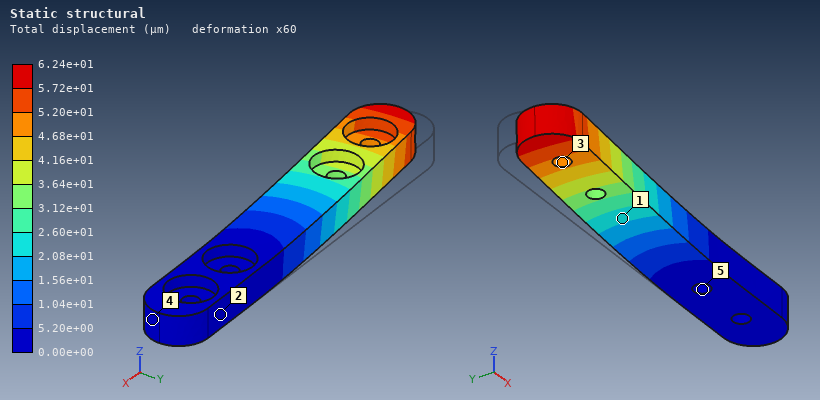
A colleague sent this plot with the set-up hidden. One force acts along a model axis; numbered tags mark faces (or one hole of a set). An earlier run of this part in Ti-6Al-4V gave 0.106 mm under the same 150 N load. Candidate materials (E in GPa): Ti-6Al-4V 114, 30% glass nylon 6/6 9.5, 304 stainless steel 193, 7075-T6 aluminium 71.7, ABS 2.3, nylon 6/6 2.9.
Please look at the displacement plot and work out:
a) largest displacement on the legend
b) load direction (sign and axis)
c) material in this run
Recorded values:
6.24e+01 µm
-Y
304 stainless steel
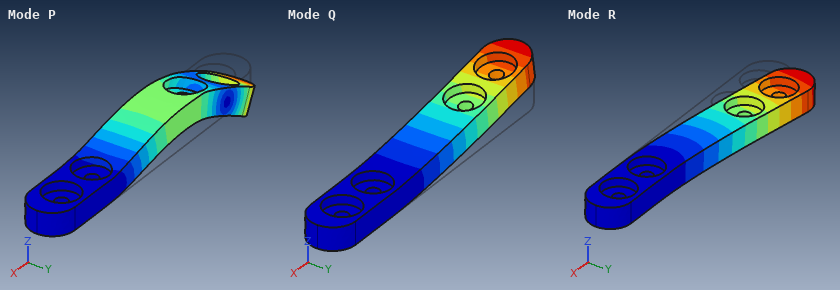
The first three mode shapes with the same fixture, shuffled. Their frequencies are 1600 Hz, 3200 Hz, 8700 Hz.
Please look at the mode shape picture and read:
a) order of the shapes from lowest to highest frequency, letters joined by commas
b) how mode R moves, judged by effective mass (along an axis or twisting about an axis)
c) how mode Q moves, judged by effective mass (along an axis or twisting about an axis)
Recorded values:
Q, R, P
along Y
along Z
